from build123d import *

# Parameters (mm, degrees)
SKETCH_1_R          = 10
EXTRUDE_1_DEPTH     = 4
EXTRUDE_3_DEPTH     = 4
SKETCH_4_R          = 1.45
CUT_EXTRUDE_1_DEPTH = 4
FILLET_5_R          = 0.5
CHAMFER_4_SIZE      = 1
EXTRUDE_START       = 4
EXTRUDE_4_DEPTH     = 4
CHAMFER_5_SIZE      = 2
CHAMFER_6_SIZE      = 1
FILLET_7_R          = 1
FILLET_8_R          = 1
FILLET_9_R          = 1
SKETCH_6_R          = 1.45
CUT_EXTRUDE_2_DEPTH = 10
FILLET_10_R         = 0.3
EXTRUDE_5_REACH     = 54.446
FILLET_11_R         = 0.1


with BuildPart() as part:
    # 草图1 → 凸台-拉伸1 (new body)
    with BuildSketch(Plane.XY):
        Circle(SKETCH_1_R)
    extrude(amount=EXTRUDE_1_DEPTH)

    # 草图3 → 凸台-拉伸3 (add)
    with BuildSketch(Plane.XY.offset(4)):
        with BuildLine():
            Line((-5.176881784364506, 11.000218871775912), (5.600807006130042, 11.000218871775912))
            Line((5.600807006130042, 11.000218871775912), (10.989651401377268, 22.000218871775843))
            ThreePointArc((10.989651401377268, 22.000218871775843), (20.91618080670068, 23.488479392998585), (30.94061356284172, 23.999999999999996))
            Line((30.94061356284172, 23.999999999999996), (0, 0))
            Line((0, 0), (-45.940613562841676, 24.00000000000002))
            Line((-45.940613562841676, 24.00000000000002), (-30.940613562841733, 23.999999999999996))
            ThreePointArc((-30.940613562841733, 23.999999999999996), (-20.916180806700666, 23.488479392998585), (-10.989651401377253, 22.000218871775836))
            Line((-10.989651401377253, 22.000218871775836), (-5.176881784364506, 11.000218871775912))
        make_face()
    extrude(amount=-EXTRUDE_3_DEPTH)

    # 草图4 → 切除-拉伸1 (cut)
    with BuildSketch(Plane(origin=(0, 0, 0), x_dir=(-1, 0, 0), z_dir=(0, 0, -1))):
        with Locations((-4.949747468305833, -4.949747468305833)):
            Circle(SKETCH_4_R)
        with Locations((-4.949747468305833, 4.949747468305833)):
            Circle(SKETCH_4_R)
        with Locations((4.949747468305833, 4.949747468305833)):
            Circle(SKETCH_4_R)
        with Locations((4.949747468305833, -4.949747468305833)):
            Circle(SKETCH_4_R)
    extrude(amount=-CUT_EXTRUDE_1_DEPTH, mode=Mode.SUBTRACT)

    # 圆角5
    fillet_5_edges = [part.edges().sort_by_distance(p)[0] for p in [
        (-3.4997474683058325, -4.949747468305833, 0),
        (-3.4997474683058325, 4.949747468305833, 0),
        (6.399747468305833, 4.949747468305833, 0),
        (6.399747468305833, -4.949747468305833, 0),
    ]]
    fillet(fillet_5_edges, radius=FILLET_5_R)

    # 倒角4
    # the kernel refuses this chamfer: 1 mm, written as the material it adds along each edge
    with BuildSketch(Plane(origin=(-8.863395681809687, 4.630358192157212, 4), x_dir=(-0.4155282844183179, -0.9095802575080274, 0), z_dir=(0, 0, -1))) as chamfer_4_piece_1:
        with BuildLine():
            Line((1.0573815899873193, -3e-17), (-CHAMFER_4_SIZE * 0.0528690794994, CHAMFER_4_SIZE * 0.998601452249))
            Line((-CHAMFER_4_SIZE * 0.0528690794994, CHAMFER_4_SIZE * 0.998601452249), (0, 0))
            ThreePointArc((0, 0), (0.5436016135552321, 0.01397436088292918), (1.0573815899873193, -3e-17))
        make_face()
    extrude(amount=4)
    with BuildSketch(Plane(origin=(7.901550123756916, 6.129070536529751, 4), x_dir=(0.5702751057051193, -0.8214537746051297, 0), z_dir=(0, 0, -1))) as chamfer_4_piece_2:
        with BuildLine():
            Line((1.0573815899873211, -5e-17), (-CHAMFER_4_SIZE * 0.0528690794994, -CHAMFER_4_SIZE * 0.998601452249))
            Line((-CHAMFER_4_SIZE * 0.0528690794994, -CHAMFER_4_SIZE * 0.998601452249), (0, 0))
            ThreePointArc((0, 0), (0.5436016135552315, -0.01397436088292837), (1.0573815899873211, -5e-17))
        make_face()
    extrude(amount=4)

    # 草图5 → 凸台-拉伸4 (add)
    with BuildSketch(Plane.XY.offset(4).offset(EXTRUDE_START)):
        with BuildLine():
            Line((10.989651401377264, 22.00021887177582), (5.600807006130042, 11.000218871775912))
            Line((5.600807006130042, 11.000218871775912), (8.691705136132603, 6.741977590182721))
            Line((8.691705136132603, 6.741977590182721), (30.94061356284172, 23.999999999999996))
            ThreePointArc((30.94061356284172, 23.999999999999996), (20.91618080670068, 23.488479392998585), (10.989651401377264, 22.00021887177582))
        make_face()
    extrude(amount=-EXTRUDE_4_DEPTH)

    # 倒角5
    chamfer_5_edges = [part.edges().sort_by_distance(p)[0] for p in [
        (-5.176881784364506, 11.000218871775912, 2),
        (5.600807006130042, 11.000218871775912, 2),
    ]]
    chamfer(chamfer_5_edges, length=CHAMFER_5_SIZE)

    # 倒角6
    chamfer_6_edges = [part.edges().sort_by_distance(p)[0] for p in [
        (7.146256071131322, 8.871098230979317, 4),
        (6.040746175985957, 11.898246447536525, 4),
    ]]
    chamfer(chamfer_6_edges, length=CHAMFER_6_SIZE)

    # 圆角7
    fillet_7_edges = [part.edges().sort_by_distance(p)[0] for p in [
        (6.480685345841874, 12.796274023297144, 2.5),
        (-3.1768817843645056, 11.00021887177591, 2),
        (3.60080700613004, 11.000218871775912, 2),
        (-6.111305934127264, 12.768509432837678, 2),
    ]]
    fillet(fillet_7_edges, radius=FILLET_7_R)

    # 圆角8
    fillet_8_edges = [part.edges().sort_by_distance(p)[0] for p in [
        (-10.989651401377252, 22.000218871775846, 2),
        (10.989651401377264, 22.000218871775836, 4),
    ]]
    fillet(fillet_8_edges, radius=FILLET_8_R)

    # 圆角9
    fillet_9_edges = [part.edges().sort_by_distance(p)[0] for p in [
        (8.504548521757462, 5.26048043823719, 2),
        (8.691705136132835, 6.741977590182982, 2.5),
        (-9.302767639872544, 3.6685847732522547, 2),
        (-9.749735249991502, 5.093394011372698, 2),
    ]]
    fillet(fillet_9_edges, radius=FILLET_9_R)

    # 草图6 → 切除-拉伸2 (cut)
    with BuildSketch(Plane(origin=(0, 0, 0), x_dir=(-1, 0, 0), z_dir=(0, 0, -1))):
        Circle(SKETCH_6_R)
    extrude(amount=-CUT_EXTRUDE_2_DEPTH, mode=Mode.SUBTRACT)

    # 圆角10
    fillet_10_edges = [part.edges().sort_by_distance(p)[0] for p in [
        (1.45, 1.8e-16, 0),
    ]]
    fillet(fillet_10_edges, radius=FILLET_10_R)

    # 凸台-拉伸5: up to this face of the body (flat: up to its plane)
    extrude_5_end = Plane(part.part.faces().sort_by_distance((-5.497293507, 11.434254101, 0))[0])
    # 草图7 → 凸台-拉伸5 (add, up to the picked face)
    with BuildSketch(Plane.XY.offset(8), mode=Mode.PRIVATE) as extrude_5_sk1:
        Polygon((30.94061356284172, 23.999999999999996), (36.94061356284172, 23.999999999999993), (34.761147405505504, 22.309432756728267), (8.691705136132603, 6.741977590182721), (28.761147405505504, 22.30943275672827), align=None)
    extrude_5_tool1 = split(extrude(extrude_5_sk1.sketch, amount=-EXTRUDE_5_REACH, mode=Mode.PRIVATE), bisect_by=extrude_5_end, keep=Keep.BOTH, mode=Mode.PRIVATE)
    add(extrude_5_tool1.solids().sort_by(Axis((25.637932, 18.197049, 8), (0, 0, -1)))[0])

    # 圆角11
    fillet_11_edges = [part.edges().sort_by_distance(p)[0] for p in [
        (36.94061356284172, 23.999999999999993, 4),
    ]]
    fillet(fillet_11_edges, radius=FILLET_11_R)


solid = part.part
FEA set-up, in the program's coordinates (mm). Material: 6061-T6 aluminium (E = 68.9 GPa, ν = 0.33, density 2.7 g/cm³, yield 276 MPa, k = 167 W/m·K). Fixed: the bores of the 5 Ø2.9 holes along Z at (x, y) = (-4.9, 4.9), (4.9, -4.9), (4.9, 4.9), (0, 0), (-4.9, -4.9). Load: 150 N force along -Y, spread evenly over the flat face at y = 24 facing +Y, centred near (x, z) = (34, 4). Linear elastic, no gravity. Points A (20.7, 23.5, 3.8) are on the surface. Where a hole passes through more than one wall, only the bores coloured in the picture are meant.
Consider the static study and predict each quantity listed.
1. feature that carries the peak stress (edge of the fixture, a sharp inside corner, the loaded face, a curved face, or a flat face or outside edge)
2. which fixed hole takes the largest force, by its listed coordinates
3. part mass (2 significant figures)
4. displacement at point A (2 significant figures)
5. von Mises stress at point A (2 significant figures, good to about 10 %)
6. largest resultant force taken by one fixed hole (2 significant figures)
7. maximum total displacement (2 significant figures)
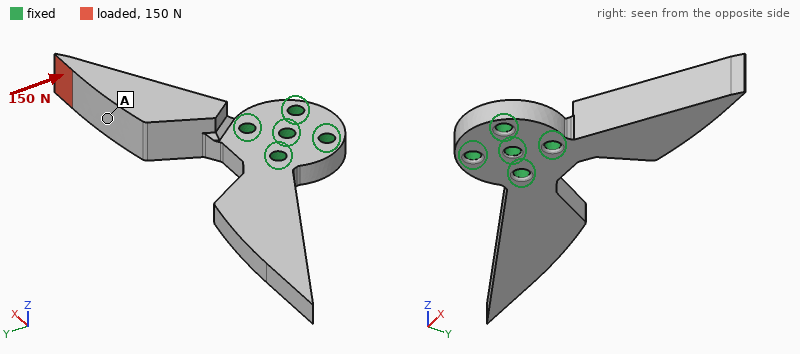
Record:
a curved face
(4.9, 4.9)
12 g
0.089 mm
19 MPa
460 N
0.17 mm
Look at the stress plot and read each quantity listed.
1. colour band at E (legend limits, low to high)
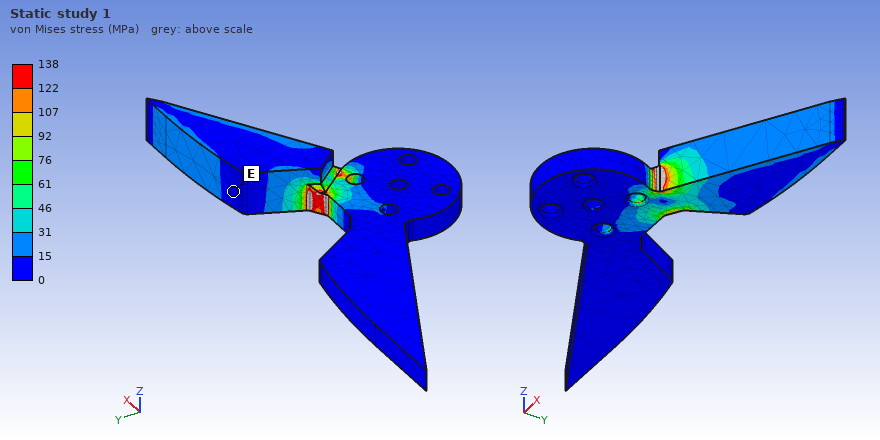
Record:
0 to 15 MPa
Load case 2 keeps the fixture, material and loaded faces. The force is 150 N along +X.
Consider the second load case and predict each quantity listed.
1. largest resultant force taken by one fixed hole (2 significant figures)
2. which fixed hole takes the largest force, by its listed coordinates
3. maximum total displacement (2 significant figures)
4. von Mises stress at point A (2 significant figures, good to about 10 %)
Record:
260 N
(-4.9, 4.9)
95 µm
9.5 MPa
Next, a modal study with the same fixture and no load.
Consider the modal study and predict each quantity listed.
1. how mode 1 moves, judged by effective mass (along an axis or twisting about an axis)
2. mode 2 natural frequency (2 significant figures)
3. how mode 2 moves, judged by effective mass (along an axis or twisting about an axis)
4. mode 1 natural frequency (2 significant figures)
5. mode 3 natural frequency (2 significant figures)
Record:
along Z
2800 Hz
along Z
2400 Hz
4100 Hz
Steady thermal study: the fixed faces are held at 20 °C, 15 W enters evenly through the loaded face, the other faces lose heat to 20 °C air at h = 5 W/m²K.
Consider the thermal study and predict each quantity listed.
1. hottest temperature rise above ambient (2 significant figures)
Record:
72 K
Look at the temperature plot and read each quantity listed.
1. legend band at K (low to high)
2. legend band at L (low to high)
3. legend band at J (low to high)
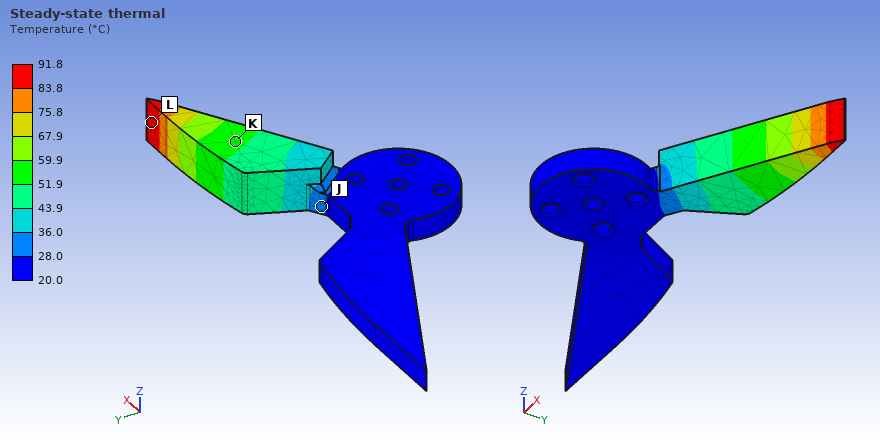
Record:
51.9 to 59.9 °C
83.8 to 91.8 °C
28.0 to 36.0 °C
